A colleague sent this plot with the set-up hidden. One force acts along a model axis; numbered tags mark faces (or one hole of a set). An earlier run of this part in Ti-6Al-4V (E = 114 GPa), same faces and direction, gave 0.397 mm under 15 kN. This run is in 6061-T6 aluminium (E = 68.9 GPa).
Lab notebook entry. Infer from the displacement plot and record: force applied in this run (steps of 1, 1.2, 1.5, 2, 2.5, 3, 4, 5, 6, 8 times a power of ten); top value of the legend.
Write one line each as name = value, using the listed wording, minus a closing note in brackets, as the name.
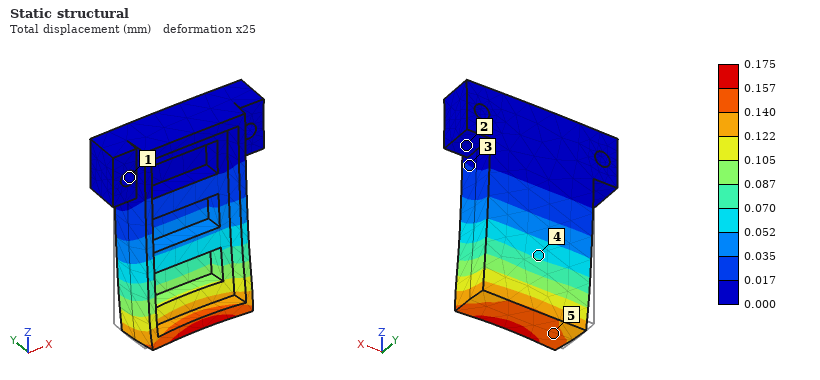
force applied in this run = 4 kN
top value of the legend = 0.175 mm
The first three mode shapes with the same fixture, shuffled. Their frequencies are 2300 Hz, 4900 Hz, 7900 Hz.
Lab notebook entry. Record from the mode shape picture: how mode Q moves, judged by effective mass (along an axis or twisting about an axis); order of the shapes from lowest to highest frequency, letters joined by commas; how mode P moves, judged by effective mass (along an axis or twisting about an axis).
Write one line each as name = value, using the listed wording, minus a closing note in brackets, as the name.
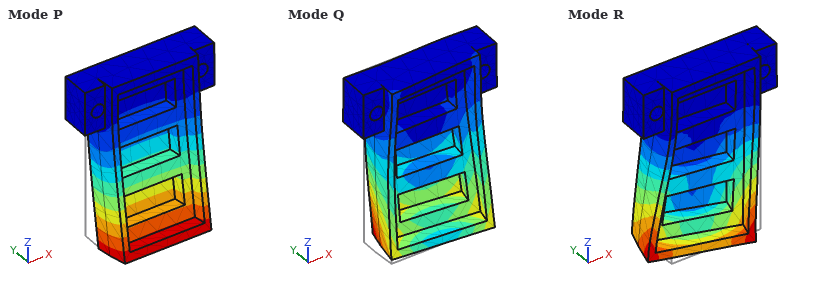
how mode Q moves, judged by effective mass = along X
order of the shapes from lowest to highest frequency, letters joined by commas = P, R, Q
how mode P moves, judged by effective mass = along Y
